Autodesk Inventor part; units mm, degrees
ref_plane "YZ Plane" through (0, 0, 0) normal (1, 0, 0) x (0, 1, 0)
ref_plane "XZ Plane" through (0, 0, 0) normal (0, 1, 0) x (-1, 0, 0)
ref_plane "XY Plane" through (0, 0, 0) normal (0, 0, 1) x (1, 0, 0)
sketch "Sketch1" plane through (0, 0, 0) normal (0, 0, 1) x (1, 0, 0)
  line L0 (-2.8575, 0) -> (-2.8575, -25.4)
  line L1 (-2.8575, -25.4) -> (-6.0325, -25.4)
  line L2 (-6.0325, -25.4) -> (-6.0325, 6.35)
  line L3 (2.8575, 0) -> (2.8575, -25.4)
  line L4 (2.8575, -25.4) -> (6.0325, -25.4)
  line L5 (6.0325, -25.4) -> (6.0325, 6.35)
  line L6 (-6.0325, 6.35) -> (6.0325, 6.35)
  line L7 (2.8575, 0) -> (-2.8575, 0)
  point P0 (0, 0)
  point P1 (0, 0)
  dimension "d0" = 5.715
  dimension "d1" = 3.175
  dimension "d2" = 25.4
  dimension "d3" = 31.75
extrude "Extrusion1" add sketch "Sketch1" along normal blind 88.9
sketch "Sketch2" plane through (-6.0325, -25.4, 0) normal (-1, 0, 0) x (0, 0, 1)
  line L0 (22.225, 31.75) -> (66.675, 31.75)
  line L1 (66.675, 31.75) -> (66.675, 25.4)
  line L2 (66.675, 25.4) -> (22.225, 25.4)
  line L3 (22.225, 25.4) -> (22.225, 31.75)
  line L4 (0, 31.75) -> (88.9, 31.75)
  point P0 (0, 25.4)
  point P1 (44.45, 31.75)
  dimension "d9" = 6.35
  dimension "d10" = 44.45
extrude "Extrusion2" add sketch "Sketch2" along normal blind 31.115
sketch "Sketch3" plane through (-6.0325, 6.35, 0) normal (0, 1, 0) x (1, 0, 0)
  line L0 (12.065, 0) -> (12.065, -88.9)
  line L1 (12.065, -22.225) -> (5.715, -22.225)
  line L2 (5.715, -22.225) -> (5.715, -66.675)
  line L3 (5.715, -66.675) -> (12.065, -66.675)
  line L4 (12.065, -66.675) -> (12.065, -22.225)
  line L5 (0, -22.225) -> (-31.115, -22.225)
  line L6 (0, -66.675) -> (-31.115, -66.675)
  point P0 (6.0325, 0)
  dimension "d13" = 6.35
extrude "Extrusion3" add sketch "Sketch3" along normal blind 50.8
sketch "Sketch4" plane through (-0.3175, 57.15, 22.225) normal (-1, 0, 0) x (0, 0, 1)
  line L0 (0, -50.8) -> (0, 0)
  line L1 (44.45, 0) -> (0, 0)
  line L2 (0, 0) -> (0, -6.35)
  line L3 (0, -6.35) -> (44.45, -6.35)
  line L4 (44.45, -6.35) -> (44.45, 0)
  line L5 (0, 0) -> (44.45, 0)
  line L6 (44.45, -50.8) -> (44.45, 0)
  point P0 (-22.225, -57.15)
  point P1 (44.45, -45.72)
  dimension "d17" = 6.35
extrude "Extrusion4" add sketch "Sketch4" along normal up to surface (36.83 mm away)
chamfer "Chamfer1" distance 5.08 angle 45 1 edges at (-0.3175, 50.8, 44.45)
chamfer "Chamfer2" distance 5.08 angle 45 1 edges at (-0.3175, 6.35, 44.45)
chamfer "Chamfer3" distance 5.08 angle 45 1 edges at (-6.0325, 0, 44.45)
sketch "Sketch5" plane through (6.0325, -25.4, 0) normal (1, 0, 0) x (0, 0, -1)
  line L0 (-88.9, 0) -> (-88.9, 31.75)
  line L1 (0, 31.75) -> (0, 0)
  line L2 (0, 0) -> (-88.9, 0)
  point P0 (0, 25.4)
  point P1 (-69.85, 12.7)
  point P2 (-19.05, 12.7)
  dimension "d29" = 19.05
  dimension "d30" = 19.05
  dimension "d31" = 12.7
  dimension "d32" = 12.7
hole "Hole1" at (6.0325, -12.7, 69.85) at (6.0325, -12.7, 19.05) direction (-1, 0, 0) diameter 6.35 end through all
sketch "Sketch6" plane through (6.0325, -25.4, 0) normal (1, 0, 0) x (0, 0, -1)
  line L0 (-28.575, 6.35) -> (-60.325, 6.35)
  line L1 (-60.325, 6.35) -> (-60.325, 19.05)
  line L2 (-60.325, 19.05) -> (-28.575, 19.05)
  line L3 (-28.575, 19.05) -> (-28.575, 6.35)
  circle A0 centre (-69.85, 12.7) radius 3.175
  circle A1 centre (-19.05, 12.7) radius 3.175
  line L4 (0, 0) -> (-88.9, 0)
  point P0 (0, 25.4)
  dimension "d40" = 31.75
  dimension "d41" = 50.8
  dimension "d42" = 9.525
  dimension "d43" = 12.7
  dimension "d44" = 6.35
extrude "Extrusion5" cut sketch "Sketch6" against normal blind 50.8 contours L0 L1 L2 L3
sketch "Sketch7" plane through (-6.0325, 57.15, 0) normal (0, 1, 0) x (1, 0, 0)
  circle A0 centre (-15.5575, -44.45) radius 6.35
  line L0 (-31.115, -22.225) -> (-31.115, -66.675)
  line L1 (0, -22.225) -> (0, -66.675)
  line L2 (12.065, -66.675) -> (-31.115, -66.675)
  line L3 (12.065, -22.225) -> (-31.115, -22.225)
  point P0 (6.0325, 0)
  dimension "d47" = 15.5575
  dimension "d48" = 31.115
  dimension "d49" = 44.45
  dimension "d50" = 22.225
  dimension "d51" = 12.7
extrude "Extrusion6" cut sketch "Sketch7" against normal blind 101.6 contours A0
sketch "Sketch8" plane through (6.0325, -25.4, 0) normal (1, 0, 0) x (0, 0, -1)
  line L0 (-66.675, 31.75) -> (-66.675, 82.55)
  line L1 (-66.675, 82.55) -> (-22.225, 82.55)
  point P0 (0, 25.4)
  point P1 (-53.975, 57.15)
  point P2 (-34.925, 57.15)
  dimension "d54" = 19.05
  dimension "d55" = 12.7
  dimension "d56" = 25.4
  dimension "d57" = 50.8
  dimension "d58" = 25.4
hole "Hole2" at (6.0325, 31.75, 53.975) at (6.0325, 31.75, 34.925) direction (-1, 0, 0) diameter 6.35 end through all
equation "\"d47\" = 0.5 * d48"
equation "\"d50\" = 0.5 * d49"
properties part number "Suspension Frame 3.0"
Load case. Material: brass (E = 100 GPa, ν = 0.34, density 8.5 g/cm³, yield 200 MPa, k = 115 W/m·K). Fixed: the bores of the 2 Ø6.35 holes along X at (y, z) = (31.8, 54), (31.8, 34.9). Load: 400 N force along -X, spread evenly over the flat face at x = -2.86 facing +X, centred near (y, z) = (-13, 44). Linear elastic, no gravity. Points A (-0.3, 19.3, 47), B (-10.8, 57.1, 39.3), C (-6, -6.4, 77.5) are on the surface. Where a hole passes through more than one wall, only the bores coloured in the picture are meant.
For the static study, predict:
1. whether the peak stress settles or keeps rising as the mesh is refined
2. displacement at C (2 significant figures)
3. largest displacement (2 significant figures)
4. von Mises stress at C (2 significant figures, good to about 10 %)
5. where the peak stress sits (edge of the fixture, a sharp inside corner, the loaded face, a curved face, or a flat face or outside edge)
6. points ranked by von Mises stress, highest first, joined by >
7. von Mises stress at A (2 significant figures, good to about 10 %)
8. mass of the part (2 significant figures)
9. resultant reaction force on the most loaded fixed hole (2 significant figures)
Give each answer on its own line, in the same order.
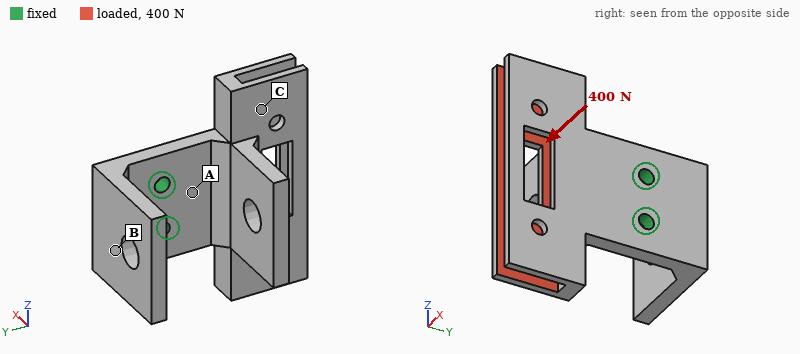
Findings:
keeps rising
0.095 mm
0.20 mm
21 MPa
edge of the fixture
A > C > B
39 MPa
440 g
200 N
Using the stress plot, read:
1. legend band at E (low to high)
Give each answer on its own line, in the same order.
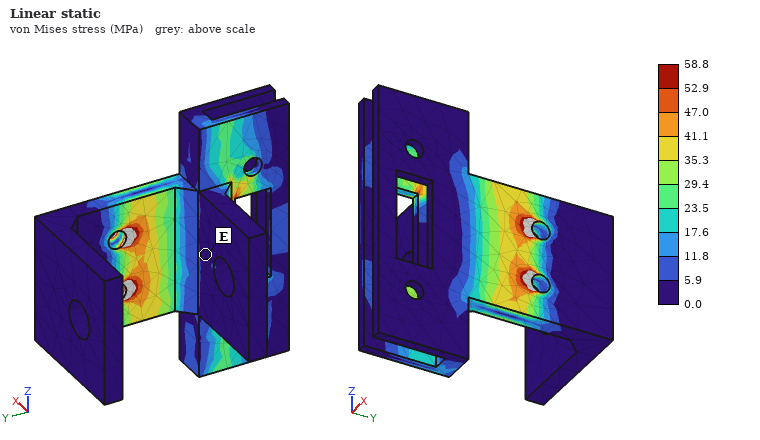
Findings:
0.0 to 5.9 MPa
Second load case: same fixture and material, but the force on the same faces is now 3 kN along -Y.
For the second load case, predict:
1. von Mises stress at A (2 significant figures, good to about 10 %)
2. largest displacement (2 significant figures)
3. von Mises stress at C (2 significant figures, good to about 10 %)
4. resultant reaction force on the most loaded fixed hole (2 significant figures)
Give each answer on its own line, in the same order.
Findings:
59 MPa
0.19 mm
25 MPa
1.5 kN
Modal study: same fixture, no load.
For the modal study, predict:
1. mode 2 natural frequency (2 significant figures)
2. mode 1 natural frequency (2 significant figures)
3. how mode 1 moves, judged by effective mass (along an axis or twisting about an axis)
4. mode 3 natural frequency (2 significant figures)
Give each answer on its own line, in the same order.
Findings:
1100 Hz
710 Hz
along X
1400 Hz
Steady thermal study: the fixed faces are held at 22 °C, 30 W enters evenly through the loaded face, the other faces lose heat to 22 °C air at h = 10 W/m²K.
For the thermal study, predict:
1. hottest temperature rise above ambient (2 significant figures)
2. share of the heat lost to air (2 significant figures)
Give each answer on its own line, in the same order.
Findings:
55 K
13 %
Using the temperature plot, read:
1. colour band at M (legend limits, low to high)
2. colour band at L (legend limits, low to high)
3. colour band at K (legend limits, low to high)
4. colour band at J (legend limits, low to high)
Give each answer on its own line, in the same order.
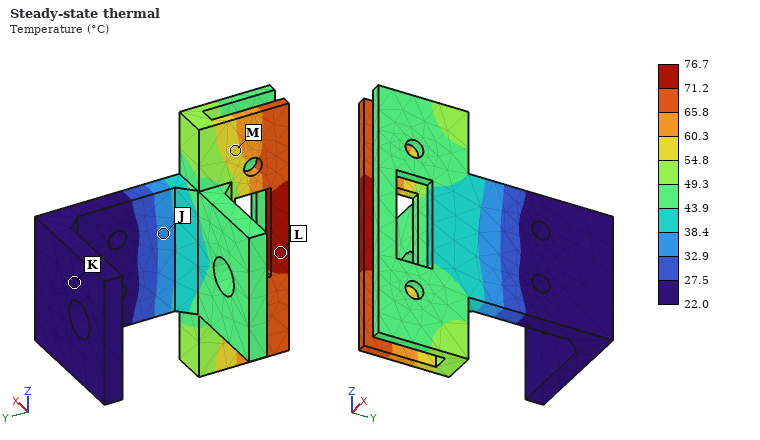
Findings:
54.8 to 60.3 °C
71.2 to 76.7 °C
22.0 to 27.5 °C
32.9 to 38.4 °C
